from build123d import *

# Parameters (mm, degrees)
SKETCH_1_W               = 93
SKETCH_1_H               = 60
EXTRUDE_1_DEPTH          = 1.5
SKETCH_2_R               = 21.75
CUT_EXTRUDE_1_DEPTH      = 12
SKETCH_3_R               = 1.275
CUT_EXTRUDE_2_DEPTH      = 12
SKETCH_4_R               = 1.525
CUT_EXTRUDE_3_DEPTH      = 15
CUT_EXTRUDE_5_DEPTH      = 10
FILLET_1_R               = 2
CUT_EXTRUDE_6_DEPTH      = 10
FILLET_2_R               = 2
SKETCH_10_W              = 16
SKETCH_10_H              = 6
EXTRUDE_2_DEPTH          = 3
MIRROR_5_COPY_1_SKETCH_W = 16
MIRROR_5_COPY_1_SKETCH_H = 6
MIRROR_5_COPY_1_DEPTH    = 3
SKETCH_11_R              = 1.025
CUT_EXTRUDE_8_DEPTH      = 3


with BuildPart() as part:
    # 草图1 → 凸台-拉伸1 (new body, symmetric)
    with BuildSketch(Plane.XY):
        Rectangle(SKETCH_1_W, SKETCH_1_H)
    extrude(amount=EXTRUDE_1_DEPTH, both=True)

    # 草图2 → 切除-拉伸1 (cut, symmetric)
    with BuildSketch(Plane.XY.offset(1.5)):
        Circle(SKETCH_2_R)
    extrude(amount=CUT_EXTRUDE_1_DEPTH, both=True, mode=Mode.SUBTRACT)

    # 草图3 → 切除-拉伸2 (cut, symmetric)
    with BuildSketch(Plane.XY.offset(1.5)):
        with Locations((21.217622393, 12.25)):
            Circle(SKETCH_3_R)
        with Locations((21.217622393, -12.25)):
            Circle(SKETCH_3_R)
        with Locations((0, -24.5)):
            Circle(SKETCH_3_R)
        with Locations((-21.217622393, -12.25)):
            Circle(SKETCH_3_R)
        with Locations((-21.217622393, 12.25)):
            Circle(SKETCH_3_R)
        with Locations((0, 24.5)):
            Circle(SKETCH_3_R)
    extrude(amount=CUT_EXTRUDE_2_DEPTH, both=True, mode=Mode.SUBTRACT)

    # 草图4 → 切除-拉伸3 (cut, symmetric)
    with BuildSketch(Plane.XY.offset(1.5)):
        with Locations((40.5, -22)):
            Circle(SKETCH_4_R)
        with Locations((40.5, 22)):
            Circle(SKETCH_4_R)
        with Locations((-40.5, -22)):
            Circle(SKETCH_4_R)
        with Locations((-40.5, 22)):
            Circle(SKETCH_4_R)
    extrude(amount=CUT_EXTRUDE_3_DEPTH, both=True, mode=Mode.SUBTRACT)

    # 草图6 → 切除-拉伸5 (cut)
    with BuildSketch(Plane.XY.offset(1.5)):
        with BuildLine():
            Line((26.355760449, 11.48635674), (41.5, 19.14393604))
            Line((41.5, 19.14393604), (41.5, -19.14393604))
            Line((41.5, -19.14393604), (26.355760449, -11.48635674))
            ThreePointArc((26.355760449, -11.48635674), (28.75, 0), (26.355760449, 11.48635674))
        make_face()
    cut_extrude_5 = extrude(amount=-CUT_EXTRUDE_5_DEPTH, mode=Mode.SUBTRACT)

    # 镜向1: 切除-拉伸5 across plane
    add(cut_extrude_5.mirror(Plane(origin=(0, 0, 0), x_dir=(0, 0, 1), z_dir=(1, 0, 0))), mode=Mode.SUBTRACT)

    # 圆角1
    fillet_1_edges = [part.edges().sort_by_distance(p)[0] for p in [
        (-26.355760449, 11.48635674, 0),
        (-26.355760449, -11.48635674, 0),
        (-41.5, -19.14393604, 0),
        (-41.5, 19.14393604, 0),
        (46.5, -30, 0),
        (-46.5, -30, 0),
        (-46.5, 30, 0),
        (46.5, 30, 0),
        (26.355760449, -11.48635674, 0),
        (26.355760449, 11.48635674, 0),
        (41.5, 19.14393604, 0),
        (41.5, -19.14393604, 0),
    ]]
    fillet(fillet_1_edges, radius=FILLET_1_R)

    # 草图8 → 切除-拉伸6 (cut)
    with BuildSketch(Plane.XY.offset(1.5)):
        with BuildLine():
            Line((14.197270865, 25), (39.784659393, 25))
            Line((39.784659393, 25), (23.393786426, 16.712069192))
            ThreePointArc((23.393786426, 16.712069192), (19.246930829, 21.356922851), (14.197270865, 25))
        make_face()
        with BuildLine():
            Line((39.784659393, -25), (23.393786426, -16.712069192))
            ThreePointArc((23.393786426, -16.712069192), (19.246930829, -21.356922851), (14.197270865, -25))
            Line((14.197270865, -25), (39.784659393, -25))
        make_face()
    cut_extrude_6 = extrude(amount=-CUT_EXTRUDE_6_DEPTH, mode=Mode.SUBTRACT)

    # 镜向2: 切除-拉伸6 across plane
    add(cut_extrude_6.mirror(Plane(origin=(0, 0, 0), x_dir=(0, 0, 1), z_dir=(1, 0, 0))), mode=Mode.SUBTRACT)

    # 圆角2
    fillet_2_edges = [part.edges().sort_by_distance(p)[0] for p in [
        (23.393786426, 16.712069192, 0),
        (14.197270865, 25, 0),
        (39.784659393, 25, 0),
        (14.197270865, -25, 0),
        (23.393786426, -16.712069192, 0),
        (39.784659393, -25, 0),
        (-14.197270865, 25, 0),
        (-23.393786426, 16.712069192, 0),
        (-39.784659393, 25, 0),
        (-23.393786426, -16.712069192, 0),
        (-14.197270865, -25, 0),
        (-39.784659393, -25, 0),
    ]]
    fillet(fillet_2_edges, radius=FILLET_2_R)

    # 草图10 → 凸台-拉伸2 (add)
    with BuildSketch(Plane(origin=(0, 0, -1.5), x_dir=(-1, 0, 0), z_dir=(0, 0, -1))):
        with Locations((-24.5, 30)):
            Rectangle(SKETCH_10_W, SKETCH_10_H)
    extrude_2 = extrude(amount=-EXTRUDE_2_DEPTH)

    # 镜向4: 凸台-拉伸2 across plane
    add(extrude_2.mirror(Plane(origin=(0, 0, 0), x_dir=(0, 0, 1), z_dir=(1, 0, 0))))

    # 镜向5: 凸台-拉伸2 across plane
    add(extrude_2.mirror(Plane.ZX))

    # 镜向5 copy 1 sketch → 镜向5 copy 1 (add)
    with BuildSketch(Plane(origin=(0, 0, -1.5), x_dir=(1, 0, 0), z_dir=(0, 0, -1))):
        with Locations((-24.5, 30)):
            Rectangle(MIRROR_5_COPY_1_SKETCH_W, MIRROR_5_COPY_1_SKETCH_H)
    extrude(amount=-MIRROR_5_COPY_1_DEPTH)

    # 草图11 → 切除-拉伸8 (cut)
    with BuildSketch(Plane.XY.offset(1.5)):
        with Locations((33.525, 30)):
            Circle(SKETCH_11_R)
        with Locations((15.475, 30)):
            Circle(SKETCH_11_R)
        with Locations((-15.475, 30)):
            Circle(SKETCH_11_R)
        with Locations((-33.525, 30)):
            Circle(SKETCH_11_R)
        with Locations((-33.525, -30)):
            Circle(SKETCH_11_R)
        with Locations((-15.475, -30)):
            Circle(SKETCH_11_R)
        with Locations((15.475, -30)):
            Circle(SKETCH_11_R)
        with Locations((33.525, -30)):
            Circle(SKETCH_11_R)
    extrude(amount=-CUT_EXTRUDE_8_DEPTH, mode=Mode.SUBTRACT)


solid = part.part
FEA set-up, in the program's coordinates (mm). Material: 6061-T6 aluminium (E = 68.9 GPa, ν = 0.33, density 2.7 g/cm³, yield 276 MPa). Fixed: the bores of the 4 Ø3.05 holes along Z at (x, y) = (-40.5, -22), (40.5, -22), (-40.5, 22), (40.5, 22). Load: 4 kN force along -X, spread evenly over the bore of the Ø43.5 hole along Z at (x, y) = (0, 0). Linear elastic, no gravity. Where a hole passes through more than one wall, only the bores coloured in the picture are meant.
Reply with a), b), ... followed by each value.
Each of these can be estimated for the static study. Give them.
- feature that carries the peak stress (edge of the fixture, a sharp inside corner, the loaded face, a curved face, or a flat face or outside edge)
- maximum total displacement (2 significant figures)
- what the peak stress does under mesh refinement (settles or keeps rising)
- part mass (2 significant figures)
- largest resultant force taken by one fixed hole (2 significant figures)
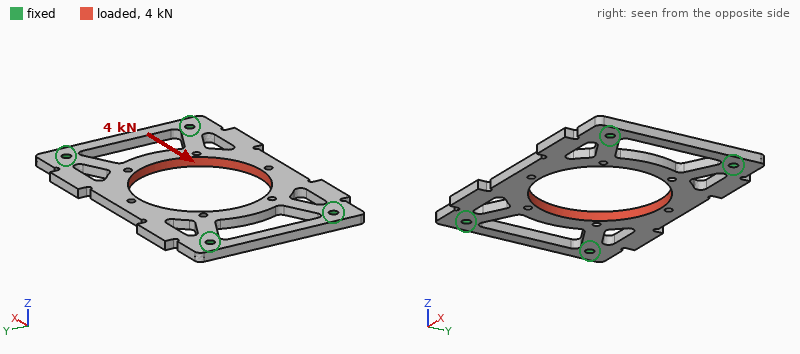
a) edge of the fixture
b) 26 µm
c) keeps rising
d) 25 g
e) 1.0 kN
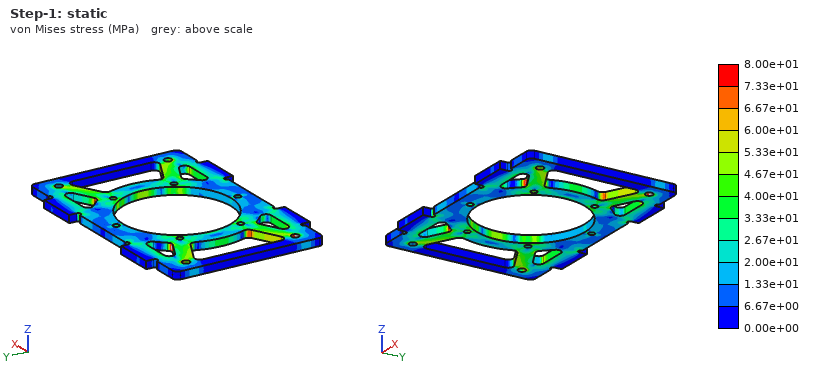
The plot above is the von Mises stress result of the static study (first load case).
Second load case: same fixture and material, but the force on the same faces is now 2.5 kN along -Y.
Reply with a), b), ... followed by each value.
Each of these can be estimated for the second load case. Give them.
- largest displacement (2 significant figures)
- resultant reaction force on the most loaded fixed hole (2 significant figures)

a) 0.10 mm
b) 640 N
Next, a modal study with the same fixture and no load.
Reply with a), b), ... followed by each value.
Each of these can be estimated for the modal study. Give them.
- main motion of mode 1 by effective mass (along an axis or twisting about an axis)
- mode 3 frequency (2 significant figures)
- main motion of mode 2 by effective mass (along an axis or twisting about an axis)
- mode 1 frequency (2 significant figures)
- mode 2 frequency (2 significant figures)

a) along Z
b) 4700 Hz
c) twisting about X
d) 2200 Hz
e) 2600 Hz
